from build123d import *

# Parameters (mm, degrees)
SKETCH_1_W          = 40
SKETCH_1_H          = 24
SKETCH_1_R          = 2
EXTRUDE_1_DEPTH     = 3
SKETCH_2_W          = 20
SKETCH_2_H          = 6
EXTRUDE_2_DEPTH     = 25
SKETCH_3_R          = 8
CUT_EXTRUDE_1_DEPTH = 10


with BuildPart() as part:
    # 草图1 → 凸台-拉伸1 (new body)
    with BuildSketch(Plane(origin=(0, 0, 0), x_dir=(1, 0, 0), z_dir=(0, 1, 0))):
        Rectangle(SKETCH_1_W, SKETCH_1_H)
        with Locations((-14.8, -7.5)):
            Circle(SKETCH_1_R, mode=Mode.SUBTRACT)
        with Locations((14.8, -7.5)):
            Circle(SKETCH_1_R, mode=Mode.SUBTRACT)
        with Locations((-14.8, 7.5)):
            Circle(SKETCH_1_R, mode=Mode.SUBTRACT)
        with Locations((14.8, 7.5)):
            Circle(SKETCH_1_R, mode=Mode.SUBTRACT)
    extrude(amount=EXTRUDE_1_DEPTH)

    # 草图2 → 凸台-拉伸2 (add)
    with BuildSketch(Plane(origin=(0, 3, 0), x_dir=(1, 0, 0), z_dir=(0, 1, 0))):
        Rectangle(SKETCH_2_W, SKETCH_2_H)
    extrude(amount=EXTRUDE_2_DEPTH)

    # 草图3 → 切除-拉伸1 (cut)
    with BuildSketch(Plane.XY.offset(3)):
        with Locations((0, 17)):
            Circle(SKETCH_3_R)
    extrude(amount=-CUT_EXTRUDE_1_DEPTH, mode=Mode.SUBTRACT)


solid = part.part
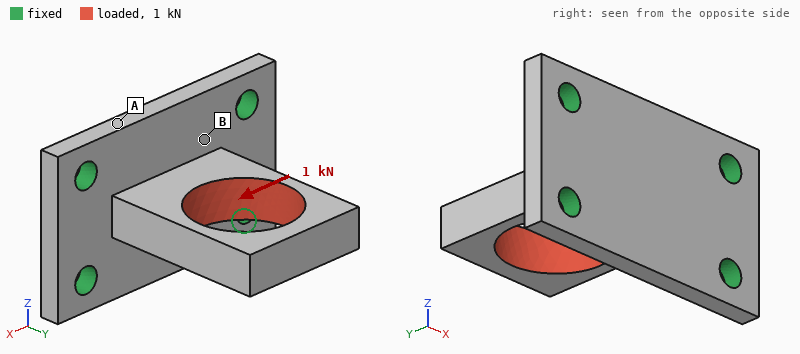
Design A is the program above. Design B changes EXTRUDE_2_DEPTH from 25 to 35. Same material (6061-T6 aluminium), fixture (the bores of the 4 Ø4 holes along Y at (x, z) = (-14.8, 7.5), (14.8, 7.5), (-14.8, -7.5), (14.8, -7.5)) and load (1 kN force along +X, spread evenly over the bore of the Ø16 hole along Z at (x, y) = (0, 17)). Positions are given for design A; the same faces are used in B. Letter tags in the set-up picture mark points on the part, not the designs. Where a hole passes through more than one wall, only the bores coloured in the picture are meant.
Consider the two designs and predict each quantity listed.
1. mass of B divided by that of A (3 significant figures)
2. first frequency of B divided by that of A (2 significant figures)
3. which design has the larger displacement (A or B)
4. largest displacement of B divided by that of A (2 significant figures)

1.27
0.44
B
1.1
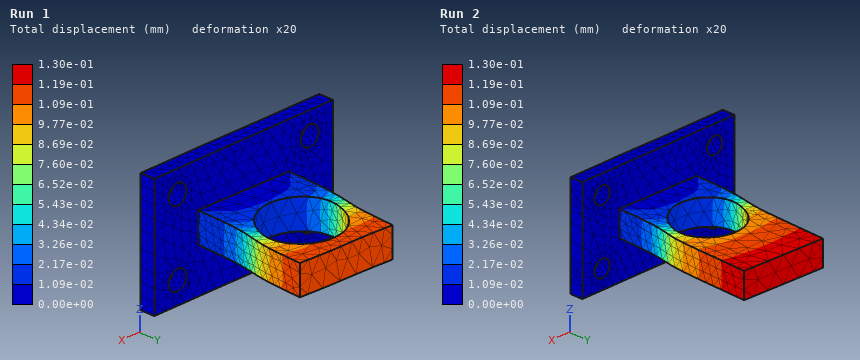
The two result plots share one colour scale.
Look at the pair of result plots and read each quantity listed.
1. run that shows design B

Run 2
